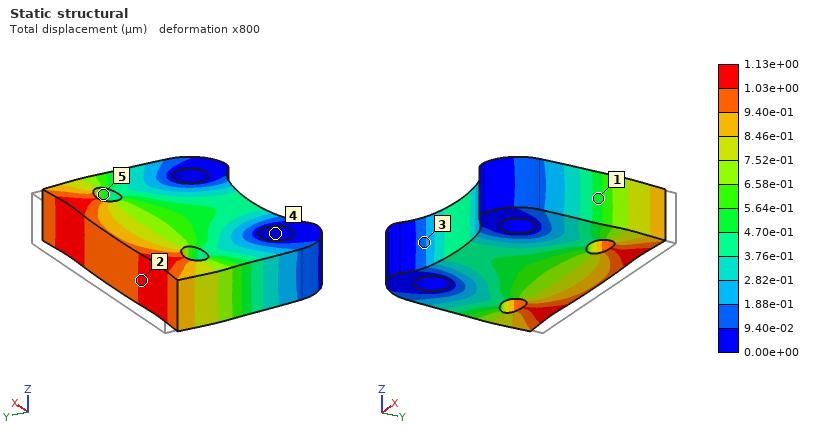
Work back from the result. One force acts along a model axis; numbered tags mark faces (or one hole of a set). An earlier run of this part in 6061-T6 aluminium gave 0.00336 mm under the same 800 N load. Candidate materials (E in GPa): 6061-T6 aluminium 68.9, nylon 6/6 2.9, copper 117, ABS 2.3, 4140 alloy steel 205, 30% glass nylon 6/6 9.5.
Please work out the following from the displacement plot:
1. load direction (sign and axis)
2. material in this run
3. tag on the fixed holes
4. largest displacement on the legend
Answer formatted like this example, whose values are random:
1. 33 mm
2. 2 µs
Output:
1. -Y
2. 4140 alloy steel
3. 4
4. 1.13e+00 µm
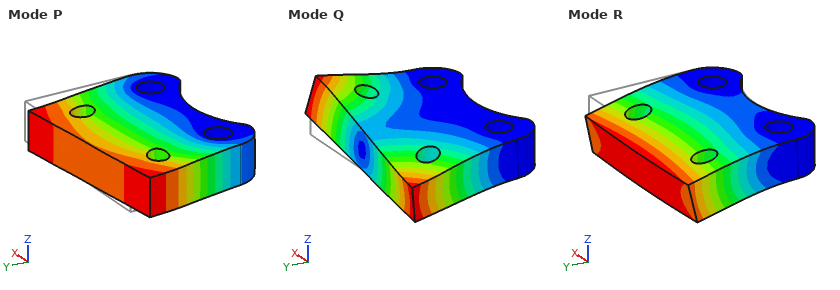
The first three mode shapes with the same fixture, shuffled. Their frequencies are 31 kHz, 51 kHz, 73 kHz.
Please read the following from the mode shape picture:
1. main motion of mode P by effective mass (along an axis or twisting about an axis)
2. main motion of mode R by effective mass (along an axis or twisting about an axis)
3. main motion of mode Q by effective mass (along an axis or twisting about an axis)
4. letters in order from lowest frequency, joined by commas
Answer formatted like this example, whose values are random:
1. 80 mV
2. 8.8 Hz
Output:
1. along X
2. along Z
3. twisting about Y
4. R, Q, P
